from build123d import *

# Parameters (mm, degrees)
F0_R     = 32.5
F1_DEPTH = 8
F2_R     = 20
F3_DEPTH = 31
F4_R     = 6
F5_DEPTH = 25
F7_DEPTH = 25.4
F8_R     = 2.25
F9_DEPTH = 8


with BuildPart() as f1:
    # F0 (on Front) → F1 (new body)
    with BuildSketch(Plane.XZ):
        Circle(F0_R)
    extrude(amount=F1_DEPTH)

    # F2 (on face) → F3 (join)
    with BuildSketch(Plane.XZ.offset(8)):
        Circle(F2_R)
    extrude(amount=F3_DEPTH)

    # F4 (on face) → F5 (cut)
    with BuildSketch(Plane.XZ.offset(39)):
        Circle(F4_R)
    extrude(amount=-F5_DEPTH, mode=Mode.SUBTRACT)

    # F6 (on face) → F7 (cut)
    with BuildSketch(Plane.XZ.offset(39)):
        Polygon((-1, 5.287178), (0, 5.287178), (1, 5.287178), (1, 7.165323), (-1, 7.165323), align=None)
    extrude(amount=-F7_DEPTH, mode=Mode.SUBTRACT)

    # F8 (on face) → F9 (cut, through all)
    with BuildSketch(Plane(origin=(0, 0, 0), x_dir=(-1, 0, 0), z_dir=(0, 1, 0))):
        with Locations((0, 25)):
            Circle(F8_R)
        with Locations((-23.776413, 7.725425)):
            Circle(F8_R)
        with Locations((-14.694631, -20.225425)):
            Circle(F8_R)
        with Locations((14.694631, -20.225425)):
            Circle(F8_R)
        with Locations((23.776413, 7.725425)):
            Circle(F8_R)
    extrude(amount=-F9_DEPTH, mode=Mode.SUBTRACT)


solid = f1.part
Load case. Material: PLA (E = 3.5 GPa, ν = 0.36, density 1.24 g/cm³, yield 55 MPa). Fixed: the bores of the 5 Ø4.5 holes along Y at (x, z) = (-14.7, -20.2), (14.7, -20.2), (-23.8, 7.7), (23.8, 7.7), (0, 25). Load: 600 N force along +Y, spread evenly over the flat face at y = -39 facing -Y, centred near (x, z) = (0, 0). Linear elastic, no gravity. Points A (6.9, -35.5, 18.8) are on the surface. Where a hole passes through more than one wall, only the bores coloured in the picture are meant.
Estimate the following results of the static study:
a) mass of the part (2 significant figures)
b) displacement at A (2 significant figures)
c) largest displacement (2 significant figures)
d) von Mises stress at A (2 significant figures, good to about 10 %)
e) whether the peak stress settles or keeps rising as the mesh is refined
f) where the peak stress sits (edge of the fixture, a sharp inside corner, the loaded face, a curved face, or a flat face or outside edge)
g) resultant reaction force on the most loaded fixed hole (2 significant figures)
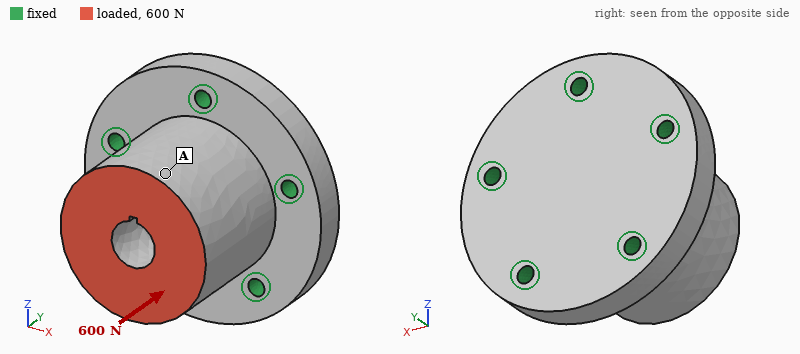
77 g
12 µm
13 µm
0.52 MPa
keeps rising
edge of the fixture
130 N
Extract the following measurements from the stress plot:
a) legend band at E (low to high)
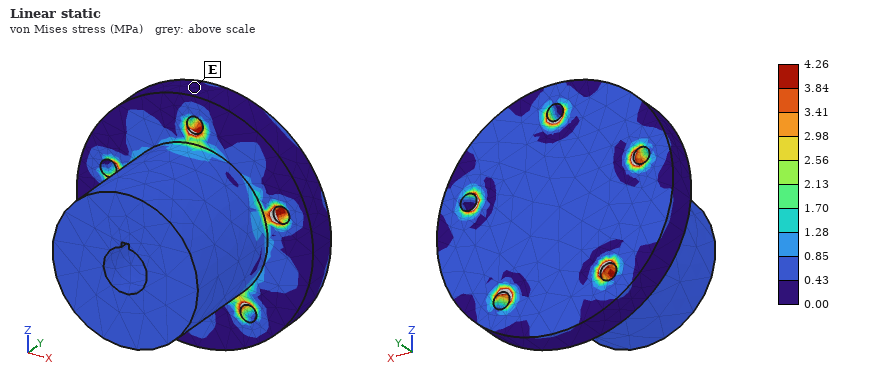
0.00 to 0.43 MPa
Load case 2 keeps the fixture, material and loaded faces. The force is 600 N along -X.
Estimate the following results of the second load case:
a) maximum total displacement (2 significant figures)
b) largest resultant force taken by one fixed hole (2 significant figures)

76 µm
380 N
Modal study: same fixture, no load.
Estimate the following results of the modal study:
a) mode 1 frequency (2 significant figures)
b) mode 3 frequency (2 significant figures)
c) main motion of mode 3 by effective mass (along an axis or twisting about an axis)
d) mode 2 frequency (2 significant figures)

3600 Hz
5300 Hz
along Y
3600 Hz
